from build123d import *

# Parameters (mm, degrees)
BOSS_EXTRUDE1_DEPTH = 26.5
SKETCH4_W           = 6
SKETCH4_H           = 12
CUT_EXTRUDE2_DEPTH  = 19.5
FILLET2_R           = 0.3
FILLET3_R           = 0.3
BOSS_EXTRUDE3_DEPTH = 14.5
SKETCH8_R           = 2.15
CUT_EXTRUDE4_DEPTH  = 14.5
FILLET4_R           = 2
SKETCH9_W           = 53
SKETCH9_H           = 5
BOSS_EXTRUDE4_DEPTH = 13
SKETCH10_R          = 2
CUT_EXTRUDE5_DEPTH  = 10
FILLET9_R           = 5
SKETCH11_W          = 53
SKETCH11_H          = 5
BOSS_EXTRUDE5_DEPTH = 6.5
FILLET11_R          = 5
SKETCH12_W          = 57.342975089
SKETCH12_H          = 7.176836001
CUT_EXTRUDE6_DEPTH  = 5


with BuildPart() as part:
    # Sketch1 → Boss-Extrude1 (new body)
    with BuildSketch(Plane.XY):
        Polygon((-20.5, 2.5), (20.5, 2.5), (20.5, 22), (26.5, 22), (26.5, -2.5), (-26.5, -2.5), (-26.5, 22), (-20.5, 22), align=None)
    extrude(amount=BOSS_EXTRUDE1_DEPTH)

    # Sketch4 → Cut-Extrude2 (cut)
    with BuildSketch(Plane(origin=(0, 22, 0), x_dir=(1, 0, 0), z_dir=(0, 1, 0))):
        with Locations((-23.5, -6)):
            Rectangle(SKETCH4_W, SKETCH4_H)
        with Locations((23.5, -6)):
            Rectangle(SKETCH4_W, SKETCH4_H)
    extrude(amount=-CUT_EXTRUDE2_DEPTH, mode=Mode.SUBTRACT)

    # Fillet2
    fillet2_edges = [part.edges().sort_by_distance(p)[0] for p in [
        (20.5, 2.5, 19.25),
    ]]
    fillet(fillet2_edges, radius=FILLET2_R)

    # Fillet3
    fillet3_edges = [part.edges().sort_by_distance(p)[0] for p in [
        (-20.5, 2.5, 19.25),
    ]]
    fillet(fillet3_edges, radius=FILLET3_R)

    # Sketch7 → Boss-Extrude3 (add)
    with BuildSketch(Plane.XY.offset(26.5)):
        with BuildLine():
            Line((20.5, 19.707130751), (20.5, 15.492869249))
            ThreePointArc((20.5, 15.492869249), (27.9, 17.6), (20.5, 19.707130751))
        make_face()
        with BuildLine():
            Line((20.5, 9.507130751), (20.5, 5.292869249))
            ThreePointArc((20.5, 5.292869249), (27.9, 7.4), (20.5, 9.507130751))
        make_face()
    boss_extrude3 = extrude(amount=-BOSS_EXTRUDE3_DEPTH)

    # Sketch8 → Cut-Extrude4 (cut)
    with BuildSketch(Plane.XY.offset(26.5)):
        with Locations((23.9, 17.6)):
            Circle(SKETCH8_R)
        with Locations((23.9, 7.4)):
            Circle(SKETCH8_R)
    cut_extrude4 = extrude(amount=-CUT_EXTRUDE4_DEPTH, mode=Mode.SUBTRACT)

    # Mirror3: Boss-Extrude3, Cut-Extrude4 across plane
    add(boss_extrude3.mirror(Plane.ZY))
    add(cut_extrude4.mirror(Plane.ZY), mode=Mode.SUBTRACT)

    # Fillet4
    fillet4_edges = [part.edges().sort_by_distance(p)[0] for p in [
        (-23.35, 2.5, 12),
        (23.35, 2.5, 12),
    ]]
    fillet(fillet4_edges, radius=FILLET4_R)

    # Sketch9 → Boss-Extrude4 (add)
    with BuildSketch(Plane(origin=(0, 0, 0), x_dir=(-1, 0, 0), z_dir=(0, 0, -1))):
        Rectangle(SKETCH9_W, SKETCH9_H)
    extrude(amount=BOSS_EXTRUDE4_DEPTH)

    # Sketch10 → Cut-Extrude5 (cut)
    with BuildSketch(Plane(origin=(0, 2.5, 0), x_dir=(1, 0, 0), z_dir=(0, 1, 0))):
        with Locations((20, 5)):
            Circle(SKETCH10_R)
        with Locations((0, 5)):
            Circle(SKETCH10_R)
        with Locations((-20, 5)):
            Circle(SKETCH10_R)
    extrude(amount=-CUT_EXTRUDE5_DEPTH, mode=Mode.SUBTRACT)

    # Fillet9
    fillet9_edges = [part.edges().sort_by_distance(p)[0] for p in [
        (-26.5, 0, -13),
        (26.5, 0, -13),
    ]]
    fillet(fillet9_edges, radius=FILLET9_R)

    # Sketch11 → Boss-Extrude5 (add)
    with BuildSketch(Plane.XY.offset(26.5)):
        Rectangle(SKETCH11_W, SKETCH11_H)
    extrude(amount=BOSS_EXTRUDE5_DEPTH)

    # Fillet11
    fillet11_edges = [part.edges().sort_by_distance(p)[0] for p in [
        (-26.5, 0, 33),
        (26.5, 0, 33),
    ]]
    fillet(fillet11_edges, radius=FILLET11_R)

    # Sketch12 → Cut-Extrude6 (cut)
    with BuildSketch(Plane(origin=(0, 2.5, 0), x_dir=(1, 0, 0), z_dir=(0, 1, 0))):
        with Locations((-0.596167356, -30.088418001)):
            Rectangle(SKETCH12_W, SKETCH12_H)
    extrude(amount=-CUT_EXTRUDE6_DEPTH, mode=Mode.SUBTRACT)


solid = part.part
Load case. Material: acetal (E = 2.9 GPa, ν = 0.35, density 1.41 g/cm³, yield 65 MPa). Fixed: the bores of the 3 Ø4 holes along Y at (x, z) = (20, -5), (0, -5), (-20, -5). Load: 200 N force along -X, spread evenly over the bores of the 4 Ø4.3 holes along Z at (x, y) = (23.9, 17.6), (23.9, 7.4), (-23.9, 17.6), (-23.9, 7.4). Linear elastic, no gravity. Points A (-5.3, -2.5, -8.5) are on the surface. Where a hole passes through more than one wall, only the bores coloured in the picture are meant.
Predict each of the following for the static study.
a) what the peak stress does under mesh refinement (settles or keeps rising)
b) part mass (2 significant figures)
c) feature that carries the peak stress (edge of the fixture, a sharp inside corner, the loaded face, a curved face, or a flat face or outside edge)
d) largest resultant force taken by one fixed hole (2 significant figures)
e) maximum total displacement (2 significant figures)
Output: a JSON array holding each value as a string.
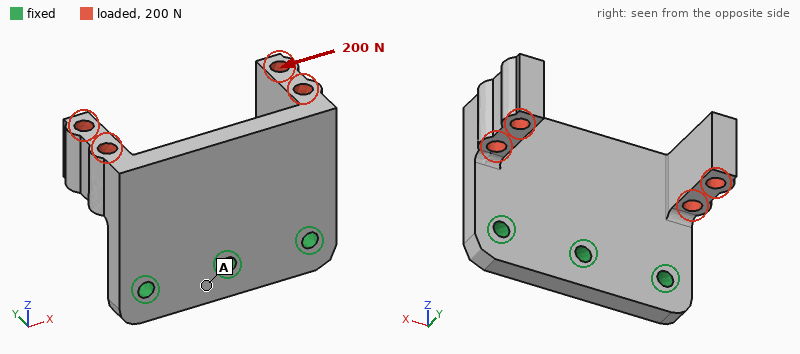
["keeps rising", "19 g", "a sharp inside corner", "140 N", "0.85 mm"]
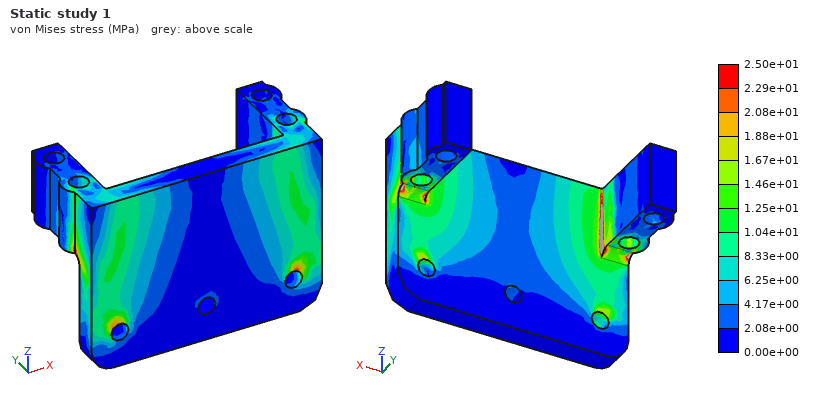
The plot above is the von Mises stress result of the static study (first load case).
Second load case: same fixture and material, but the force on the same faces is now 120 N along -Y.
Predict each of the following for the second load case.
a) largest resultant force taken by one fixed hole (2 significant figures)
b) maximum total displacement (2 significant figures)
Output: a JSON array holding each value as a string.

["49 N", "0.76 mm"]
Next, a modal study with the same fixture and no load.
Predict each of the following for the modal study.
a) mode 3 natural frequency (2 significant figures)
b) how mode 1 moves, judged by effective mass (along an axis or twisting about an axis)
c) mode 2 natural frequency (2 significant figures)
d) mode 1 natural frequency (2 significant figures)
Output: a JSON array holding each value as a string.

["1500 Hz", "along Y", "1000 Hz", "800 Hz"]
